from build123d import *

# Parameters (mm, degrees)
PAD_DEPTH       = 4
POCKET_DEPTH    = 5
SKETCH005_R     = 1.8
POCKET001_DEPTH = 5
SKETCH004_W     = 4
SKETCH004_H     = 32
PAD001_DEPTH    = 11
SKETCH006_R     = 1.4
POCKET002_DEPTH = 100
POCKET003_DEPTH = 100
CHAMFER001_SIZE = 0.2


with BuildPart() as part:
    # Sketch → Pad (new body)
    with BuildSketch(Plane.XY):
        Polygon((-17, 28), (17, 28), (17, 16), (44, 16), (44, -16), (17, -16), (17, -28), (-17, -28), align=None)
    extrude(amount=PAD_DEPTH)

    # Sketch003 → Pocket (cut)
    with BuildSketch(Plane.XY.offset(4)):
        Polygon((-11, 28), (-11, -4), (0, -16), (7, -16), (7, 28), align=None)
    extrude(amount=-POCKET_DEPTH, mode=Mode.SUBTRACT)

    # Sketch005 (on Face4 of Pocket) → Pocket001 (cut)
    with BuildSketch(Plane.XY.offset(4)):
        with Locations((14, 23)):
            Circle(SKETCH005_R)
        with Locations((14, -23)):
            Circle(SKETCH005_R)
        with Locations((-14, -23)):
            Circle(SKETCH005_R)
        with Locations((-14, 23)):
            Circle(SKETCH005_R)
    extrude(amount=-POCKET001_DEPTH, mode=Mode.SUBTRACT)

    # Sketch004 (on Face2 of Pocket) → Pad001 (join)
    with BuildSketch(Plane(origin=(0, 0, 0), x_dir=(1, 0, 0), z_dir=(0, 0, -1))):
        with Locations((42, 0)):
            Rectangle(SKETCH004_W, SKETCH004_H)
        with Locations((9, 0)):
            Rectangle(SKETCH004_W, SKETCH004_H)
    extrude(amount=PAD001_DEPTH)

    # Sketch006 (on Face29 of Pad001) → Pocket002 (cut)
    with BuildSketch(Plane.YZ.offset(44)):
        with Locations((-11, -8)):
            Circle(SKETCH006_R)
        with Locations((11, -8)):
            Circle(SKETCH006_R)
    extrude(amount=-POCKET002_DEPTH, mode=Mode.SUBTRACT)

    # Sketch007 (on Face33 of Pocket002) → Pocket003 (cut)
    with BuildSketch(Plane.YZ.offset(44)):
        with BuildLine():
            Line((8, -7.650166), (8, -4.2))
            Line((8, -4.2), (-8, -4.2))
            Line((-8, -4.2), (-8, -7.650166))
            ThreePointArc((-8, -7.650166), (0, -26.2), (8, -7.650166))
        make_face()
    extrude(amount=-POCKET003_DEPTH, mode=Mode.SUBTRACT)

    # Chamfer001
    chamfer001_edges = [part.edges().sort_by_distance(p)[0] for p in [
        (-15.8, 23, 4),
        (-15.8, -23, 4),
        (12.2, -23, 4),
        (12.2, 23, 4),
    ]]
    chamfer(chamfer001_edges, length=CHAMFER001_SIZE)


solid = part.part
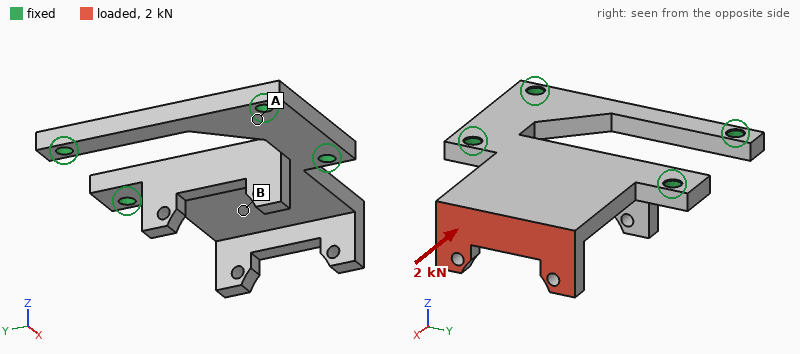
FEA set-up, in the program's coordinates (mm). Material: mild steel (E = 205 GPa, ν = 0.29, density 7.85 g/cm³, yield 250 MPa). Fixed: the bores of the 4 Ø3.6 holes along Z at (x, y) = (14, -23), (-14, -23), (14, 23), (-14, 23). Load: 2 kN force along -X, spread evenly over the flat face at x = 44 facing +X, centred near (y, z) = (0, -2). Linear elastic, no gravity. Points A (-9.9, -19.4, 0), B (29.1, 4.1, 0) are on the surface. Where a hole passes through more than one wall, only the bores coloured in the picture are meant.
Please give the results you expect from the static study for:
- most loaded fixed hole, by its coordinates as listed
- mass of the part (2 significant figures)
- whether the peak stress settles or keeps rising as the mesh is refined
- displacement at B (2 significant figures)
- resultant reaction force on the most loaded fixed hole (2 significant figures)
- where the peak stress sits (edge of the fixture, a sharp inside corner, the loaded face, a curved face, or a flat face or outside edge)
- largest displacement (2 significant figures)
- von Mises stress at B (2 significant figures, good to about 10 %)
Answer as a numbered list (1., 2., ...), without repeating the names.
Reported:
1. (14, 23)
2. 77 g
3. keeps rising
4. 0.070 mm
5. 940 N
6. edge of the fixture
7. 0.22 mm
8. 97 MPa
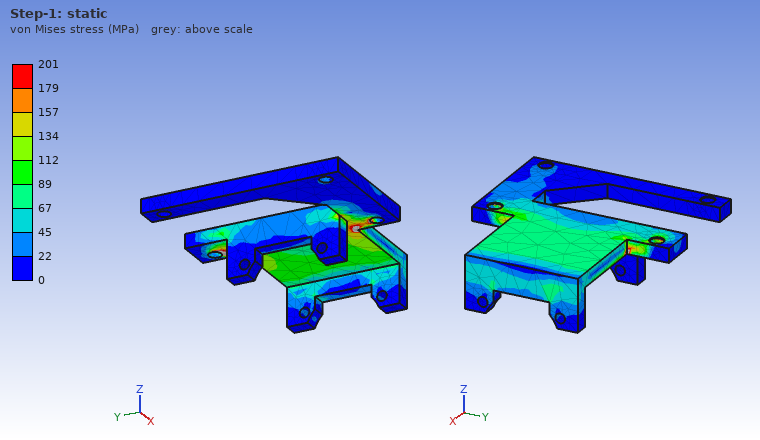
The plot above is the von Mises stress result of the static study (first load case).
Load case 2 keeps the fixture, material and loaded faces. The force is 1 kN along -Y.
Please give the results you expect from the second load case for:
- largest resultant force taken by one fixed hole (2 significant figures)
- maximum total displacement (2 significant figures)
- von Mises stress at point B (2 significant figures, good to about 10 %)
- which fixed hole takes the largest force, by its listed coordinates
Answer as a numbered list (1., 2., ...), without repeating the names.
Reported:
1. 930 N
2. 44 µm
3. 51 MPa
4. (14, 23)
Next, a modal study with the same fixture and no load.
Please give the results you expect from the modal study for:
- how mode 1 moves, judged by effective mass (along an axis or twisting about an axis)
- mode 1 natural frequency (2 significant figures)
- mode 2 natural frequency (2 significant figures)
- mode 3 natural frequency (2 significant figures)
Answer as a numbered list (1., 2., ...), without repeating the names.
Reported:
1. along Z
2. 1700 Hz
3. 5200 Hz
4. 9000 Hz
